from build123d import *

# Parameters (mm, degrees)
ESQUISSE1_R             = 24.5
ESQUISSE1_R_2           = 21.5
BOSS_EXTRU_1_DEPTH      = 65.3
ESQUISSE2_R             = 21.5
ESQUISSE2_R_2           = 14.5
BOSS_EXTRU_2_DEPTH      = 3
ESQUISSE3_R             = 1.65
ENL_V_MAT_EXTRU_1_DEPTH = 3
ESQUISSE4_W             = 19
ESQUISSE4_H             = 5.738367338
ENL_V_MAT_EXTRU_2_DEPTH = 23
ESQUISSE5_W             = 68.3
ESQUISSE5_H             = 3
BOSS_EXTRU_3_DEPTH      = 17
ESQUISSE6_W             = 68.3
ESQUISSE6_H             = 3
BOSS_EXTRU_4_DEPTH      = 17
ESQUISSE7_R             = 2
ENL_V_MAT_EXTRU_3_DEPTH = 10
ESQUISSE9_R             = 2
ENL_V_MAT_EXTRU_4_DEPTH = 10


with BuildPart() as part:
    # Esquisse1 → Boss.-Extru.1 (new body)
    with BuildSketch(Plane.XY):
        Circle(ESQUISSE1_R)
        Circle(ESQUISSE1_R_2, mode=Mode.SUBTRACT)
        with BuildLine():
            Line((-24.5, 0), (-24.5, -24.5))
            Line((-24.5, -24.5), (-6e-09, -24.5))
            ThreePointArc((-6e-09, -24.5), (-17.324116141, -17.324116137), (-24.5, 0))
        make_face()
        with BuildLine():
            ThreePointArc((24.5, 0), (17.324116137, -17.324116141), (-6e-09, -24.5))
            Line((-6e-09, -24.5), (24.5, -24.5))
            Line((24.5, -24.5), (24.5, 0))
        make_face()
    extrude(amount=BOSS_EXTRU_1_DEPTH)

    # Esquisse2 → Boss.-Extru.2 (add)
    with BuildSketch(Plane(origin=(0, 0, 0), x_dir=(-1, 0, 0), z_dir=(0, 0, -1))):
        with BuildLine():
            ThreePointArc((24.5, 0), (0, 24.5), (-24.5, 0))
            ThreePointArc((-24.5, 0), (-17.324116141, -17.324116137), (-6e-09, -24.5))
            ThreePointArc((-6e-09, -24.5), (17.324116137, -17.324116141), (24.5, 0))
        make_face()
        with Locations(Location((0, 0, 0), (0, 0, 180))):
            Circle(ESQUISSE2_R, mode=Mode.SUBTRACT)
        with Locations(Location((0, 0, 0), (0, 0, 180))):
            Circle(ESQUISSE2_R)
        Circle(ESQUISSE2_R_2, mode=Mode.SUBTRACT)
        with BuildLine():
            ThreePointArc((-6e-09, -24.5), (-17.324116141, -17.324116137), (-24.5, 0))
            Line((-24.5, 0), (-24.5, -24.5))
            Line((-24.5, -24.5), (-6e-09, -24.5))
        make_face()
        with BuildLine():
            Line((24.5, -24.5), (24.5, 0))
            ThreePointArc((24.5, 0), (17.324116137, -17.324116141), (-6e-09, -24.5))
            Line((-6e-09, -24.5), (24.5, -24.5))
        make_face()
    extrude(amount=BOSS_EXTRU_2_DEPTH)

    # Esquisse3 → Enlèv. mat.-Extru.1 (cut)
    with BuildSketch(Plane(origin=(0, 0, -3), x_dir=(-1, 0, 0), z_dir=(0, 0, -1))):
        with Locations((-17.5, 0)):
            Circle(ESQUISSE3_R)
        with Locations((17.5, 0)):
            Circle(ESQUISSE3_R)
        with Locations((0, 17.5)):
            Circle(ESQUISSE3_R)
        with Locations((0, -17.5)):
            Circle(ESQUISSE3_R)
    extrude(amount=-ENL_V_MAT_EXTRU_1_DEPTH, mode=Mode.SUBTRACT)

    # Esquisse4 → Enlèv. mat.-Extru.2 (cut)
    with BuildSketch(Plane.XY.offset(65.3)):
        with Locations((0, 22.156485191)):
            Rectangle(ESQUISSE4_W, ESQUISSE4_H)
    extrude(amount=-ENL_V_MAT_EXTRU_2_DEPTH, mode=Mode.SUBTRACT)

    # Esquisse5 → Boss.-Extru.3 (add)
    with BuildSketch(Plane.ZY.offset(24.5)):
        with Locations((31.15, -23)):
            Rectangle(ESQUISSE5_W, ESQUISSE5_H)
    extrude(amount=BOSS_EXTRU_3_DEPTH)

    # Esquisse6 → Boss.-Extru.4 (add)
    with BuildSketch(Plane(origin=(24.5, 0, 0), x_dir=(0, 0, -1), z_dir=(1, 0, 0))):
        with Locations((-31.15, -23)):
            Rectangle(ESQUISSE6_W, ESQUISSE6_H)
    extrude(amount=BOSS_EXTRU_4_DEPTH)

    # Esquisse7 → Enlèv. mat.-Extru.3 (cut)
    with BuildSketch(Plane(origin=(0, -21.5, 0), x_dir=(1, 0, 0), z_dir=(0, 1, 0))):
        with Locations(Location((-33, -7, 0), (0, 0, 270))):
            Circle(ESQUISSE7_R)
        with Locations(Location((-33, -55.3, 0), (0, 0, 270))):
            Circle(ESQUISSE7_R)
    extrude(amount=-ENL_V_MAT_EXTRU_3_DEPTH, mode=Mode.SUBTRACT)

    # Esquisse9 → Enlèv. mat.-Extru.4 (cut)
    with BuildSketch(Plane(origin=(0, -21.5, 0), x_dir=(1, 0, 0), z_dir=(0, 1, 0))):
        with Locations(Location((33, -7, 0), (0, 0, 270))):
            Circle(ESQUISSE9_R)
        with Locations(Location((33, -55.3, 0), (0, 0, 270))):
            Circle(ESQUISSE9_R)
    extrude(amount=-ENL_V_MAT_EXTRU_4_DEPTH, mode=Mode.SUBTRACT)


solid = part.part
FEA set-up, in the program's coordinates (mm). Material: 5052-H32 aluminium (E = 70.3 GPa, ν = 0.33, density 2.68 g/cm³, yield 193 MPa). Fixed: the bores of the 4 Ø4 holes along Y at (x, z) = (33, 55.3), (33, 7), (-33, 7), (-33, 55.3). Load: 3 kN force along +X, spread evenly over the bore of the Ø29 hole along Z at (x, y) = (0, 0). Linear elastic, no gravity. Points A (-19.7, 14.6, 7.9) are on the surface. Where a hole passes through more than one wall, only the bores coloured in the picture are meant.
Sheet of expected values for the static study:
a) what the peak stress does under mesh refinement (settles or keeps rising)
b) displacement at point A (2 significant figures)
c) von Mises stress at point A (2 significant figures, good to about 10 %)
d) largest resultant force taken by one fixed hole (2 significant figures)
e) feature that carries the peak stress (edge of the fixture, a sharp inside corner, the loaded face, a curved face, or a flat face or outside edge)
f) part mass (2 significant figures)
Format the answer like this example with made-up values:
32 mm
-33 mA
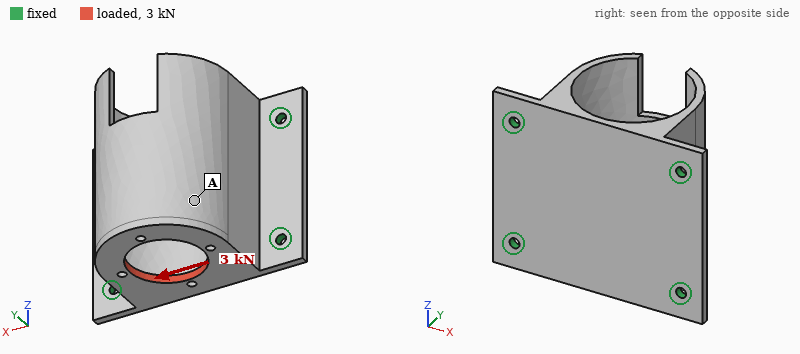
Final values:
keeps rising
82 µm
14 MPa
1.4 kN
edge of the fixture
150 g
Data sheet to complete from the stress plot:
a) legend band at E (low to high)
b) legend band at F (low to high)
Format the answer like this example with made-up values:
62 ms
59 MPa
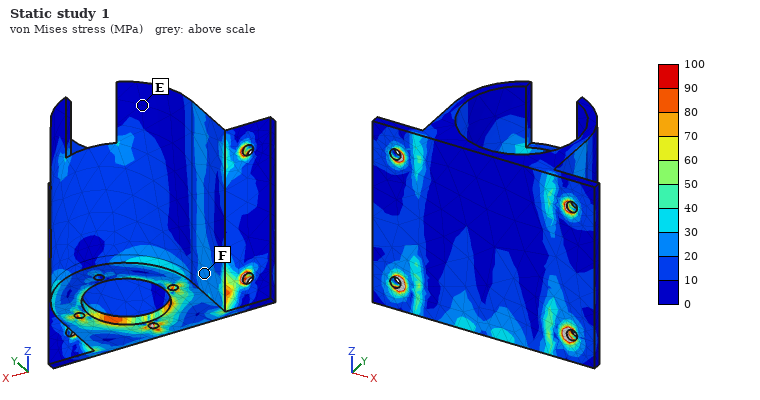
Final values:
0 to 10 MPa
20 to 30 MPa
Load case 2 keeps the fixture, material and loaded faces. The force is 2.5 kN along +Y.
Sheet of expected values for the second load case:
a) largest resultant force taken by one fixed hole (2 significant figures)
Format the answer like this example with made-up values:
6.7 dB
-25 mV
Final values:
1.6 kN
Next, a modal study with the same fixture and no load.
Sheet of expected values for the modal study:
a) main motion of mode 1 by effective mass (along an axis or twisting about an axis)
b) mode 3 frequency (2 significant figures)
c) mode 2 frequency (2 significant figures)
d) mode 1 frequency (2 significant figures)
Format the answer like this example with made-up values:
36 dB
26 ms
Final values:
along X
3600 Hz
3500 Hz
3100 Hz
